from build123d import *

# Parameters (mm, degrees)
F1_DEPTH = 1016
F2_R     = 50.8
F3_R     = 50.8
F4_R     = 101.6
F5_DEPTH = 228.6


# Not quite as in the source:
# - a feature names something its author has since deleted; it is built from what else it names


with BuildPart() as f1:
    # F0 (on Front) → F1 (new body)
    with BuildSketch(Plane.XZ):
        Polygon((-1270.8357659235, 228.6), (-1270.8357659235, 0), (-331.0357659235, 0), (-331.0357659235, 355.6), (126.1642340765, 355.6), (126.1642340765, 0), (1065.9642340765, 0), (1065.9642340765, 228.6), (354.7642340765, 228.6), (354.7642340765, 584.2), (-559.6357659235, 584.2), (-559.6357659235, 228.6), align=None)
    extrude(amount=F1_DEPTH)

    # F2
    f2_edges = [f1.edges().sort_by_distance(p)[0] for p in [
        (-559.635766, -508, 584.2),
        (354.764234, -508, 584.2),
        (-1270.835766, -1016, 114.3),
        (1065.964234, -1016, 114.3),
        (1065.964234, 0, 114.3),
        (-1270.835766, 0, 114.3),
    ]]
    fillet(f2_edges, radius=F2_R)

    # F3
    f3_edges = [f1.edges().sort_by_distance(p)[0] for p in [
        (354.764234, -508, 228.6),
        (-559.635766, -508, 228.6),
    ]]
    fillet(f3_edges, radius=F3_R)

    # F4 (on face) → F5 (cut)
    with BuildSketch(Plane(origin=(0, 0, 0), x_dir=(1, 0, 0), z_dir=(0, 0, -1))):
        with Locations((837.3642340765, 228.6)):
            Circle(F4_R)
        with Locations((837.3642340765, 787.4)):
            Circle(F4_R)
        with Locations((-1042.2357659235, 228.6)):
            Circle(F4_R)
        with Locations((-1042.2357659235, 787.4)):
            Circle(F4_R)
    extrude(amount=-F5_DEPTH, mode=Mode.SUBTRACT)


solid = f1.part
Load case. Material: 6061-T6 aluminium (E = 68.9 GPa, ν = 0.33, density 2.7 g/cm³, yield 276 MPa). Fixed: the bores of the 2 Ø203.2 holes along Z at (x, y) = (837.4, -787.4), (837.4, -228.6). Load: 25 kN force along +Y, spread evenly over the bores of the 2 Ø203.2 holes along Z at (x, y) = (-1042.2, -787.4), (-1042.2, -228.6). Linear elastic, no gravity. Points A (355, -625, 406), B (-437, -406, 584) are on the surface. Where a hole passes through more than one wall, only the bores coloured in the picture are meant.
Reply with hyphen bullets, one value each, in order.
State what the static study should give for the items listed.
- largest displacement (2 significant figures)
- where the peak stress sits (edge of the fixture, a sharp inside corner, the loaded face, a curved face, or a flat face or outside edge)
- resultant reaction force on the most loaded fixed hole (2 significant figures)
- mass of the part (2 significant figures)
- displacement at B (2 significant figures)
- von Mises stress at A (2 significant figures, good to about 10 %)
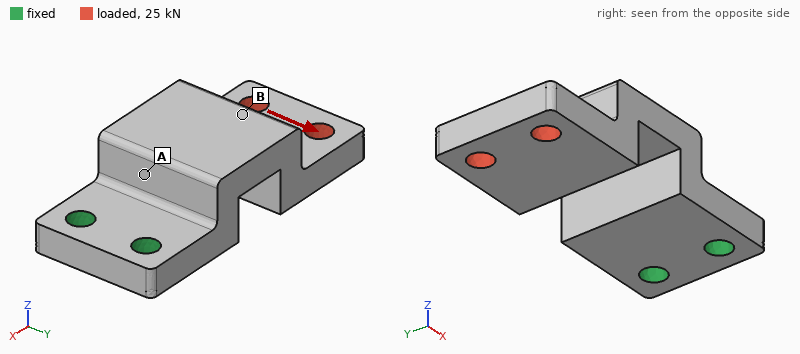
- 0.18 mm
- a curved face
- 69 kN
- 1800 kg
- 0.043 mm
- 1.5 MPa
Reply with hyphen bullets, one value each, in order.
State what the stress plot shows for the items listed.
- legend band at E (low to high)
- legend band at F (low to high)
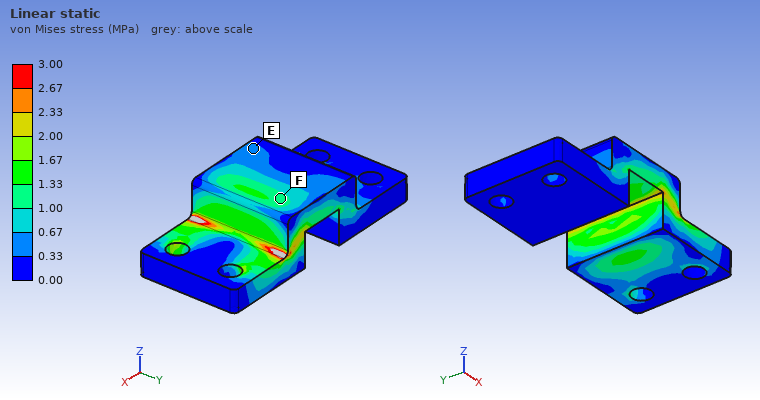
- 0.33 to 0.67 MPa
- 1.00 to 1.33 MPa
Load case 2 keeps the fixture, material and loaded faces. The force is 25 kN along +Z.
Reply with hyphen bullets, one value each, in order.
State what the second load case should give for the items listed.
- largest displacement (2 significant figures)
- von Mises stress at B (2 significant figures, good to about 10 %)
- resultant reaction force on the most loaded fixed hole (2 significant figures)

- 1.0 mm
- 0.73 MPa
- 13 kN
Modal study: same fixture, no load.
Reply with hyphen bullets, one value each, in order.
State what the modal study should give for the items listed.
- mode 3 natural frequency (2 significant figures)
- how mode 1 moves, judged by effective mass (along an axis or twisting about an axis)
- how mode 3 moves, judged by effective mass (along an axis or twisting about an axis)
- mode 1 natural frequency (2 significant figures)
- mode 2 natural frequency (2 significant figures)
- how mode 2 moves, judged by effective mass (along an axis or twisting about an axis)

- 150 Hz
- along Z
- along X
- 39 Hz
- 93 Hz
- along Y
